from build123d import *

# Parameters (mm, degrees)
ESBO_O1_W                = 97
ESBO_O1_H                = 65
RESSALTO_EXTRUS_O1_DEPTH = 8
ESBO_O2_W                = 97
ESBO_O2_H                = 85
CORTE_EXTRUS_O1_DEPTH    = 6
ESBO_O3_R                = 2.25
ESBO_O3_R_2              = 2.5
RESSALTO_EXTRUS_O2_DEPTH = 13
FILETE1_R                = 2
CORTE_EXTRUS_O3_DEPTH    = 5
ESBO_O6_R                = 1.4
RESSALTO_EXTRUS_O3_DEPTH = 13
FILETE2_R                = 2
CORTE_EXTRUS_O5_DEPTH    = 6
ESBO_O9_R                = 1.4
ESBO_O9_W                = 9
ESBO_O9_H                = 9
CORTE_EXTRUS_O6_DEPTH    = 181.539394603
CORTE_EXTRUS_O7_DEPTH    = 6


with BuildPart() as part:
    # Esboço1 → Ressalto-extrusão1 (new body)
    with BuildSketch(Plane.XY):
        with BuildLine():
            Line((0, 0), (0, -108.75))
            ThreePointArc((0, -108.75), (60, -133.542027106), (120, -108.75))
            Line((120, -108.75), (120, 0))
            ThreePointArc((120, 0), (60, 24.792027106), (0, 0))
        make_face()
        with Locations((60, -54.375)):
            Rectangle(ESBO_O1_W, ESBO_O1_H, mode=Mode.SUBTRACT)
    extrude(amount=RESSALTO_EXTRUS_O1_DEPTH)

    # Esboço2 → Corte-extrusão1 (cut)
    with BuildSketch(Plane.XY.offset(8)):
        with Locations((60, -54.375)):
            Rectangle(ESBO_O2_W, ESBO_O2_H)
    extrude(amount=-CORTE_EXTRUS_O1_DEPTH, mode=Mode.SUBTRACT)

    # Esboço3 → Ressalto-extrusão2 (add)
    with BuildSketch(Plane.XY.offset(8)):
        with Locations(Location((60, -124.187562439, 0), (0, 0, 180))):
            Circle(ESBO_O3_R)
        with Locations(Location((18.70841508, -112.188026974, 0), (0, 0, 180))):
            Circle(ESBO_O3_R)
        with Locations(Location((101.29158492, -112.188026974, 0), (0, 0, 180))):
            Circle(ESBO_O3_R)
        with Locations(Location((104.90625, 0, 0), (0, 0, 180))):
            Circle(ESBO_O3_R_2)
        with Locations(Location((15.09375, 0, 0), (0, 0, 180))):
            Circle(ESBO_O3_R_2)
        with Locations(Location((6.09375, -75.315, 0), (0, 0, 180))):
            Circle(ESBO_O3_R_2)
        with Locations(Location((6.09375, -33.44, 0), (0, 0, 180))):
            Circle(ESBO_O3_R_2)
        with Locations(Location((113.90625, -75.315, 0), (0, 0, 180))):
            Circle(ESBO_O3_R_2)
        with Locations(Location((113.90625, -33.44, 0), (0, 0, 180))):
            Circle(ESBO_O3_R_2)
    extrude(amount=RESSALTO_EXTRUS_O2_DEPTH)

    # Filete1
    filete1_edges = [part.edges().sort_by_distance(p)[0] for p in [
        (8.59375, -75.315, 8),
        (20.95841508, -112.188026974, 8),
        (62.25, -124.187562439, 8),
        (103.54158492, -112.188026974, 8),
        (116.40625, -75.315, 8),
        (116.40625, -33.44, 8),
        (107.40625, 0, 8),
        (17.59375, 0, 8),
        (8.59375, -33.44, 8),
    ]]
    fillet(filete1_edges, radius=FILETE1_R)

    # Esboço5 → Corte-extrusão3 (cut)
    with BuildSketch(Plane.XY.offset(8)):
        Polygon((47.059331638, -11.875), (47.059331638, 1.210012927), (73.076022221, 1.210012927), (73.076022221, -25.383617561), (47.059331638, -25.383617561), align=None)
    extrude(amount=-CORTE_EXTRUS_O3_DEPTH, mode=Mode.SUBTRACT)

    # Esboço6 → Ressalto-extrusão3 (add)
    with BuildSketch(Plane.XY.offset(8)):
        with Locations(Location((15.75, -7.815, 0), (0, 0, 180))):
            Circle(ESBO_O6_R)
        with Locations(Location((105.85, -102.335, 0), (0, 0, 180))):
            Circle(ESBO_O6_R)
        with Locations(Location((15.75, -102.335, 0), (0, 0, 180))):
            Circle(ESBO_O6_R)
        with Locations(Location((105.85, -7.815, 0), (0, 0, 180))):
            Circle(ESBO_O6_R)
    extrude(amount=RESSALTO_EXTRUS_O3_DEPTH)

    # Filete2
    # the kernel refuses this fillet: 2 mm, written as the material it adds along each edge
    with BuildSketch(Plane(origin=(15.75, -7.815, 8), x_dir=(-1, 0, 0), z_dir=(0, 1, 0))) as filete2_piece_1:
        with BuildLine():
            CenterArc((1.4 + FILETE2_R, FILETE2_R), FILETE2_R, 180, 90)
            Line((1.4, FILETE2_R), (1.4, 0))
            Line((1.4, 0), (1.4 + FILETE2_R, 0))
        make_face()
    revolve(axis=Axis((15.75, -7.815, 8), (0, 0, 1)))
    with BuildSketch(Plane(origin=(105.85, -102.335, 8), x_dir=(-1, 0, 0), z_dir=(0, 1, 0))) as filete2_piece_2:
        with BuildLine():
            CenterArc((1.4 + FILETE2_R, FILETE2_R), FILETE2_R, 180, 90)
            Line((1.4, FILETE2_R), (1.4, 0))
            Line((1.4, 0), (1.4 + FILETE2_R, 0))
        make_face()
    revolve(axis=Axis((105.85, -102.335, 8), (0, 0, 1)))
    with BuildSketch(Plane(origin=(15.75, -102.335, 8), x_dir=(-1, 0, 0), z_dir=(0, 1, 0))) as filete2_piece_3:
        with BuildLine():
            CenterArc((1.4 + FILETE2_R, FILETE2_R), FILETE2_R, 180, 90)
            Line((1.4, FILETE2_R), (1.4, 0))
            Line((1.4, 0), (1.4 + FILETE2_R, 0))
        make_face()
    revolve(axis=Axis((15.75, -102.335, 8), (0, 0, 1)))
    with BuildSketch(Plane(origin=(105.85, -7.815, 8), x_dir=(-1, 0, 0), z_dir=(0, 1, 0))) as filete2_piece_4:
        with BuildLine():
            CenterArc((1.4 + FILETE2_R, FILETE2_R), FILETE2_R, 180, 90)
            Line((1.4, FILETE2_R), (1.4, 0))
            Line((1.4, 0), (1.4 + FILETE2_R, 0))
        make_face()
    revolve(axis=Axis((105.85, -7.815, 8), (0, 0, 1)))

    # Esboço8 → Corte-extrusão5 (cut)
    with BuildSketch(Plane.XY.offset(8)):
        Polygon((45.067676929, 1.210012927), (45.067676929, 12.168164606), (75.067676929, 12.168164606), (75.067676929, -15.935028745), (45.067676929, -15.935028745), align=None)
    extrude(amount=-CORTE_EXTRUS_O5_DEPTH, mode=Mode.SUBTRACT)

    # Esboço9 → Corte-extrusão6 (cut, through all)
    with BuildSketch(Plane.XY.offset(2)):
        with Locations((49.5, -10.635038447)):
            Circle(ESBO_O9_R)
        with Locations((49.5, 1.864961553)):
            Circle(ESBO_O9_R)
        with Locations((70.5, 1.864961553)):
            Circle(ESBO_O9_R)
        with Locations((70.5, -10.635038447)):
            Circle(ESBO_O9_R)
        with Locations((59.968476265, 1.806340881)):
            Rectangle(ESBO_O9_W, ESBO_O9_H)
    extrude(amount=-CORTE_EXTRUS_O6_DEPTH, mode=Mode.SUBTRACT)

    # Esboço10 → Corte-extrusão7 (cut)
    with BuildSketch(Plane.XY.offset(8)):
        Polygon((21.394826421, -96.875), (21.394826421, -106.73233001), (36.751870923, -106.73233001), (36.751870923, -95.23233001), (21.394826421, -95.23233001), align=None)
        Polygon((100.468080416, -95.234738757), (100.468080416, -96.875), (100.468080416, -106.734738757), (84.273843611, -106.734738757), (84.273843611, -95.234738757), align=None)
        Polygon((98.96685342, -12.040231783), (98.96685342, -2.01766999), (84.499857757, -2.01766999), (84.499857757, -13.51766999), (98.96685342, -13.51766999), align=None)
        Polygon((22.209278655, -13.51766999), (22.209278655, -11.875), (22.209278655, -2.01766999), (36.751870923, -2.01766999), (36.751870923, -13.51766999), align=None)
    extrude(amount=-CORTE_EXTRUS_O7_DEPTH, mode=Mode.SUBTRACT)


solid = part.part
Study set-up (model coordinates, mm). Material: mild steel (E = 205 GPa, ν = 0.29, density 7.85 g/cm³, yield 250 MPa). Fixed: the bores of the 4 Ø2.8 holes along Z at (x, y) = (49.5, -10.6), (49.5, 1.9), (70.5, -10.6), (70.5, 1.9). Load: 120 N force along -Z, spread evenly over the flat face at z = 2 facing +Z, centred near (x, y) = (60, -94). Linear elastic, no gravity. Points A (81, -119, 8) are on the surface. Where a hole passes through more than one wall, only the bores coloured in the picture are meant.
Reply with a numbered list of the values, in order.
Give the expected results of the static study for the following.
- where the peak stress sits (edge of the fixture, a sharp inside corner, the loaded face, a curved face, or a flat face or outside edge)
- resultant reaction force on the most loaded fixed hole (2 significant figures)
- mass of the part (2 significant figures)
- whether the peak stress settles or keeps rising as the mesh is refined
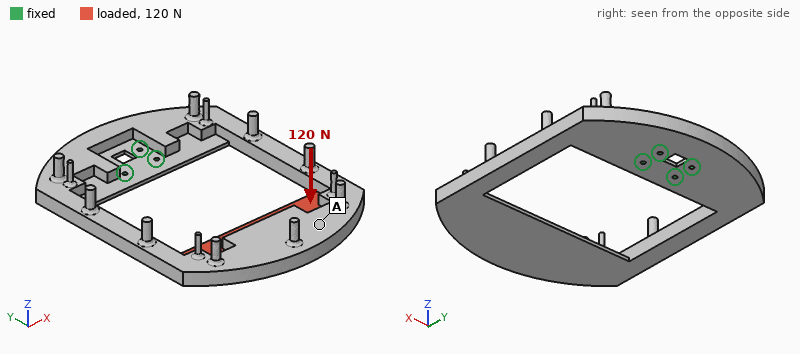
1. edge of the fixture
2. 430 N
3. 550 g
4. keeps rising
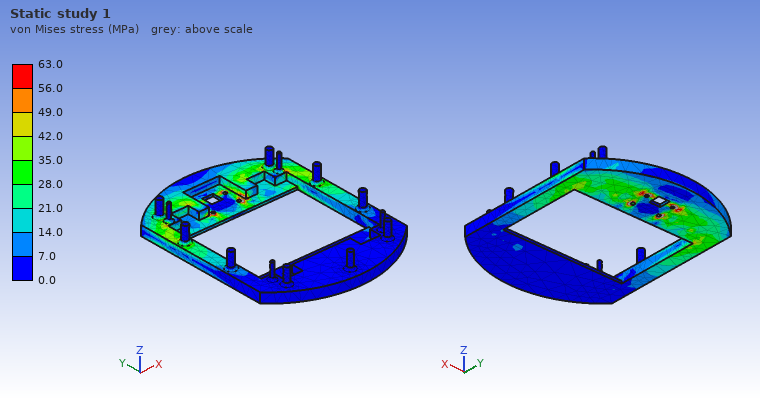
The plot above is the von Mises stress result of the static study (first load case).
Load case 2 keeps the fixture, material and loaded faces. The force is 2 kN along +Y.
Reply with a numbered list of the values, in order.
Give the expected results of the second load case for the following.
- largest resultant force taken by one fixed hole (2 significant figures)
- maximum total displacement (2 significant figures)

1. 890 N
2. 0.20 mm
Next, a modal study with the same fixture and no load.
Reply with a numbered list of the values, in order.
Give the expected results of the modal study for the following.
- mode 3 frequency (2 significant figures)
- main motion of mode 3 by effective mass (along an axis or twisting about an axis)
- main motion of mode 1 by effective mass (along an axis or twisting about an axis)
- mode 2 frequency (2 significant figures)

1. 660 Hz
2. along X
3. along Z
4. 420 Hz
